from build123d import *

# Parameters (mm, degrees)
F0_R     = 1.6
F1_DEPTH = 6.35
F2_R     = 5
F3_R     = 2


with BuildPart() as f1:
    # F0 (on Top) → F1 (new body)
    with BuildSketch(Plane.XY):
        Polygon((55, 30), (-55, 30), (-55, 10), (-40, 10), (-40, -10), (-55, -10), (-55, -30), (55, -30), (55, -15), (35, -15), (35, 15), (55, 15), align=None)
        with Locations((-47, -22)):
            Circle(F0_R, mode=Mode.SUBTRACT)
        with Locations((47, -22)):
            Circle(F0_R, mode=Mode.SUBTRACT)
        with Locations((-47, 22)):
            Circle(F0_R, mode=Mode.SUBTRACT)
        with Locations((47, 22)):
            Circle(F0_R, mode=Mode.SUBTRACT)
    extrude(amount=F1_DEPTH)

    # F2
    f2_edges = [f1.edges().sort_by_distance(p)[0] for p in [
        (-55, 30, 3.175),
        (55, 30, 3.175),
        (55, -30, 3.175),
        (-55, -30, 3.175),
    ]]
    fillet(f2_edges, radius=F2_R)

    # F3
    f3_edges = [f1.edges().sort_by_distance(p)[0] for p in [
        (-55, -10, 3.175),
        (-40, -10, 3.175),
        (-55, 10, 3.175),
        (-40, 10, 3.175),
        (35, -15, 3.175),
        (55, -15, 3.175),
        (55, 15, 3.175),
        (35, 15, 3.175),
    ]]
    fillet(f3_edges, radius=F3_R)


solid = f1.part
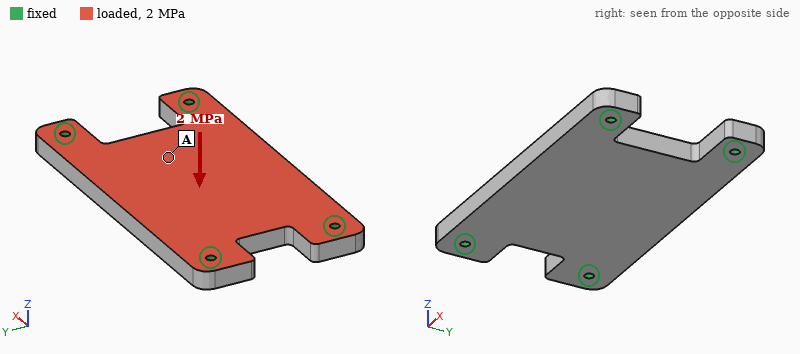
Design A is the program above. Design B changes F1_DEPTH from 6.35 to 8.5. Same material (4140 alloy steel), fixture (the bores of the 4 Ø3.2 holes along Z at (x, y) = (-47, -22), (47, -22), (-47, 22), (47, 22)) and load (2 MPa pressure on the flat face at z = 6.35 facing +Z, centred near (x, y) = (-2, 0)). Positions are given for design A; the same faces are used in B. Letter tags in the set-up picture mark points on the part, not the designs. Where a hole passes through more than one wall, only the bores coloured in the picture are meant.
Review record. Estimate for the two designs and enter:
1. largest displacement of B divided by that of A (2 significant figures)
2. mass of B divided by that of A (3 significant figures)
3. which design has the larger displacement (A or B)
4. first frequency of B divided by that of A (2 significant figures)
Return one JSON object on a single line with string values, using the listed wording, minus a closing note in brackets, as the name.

{"largest displacement of B divided by that of A": "0.45", "mass of B divided by that of A": "1.34", "which design has the larger displacement": "A", "first frequency of B divided by that of A": "1.3"}
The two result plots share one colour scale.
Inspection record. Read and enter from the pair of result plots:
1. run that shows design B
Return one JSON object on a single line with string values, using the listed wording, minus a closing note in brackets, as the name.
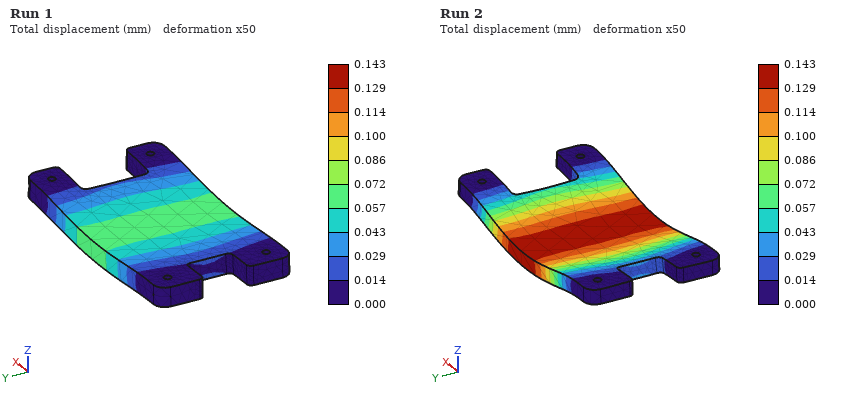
{"run that shows design B": "Run 1"}
